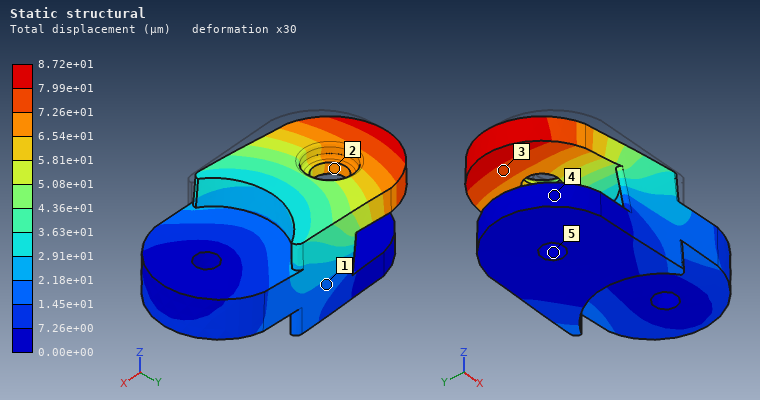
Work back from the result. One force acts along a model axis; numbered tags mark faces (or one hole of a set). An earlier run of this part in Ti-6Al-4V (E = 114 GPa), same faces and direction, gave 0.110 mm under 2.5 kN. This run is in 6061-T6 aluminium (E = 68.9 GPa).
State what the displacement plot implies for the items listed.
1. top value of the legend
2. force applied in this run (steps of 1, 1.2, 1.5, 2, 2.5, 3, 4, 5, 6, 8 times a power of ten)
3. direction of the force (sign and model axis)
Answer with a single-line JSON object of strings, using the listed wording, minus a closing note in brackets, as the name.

{"top value of the legend": "8.72e+01 µm", "force applied in this run": "1.2 kN", "direction of the force": "+Y"}
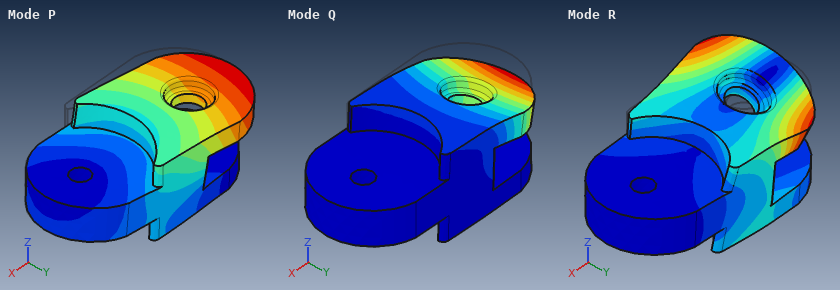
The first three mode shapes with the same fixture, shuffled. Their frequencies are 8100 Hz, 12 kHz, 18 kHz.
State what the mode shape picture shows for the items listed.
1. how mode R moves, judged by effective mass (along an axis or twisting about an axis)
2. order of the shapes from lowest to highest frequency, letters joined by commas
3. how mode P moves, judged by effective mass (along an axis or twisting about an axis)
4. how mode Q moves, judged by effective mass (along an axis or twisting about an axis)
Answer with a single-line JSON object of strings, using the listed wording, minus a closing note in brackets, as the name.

{"how mode R moves, judged by effective mass": "twisting about X", "order of the shapes from lowest to highest frequency, letters joined by commas": "Q, P, R", "how mode P moves, judged by effective mass": "along Y", "how mode Q moves, judged by effective mass": "along Z"}
